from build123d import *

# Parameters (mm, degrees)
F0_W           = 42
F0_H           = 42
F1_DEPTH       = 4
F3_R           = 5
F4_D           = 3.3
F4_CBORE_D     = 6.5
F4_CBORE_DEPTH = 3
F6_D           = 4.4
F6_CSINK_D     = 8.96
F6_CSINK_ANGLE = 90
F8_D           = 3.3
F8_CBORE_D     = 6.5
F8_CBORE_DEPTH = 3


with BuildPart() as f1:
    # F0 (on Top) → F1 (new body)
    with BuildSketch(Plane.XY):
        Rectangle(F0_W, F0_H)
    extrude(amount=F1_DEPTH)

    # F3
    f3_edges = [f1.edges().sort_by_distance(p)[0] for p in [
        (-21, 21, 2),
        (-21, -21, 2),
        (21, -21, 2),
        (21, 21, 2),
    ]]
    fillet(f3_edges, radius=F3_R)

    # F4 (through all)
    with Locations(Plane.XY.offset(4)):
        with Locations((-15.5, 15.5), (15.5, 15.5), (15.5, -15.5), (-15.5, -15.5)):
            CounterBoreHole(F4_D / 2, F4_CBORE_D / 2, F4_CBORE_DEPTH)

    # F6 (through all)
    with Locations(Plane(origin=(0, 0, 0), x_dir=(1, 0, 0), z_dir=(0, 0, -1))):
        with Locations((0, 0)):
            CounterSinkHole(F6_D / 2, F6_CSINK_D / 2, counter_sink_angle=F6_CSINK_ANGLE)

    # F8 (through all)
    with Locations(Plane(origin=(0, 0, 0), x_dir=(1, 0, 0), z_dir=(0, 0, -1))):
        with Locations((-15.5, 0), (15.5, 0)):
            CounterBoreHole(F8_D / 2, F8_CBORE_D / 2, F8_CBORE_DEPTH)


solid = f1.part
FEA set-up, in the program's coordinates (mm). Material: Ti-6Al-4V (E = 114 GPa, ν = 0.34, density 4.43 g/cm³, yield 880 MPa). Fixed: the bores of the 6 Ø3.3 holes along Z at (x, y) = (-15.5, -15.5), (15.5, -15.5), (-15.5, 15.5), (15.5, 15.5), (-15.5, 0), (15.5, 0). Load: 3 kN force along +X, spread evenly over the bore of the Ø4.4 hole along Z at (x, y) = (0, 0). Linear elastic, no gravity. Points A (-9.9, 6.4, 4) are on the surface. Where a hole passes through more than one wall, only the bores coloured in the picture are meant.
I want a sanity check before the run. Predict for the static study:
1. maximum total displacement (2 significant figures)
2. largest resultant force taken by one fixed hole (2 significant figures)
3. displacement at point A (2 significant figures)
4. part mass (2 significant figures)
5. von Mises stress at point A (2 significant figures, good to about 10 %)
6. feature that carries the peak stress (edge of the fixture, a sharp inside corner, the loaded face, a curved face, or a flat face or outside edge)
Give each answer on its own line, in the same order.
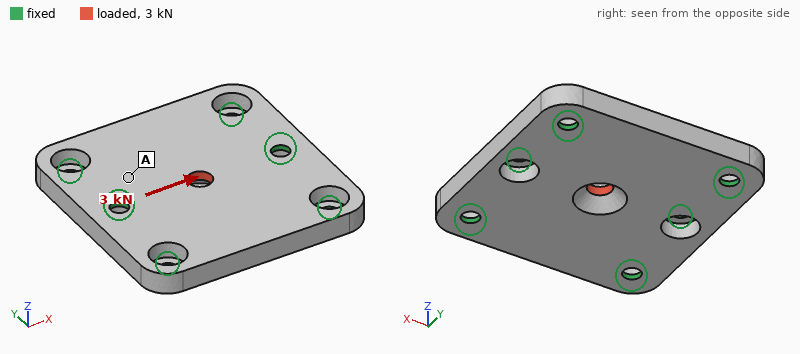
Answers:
7.8 µm
700 N
2.4 µm
28 g
18 MPa
the loaded face
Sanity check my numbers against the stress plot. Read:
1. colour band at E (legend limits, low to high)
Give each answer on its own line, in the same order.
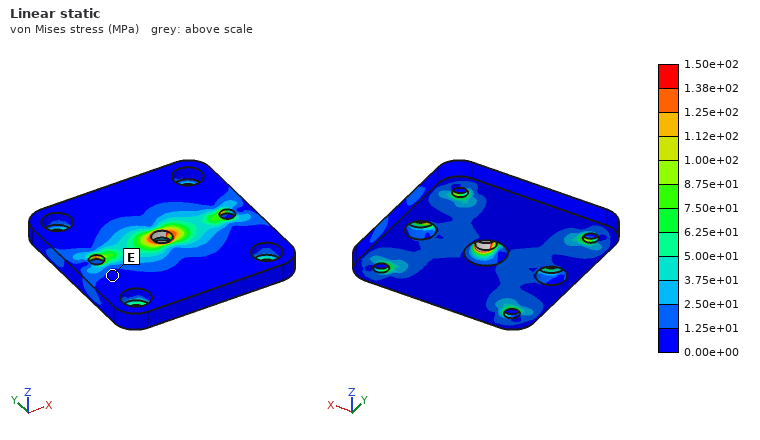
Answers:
0.00e+00 to 1.25e+01 MPa
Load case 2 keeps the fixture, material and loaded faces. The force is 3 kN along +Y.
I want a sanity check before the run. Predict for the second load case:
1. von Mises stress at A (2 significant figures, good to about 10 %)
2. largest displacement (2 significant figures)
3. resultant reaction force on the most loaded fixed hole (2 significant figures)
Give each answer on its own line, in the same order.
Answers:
24 MPa
9.3 µm
610 N
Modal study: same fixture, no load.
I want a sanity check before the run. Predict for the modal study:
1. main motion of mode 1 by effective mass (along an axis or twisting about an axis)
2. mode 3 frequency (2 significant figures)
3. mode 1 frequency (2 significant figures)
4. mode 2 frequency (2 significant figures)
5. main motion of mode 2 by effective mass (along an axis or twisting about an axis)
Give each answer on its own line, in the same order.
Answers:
along Z
22 kHz
13 kHz
15 kHz
twisting about X
